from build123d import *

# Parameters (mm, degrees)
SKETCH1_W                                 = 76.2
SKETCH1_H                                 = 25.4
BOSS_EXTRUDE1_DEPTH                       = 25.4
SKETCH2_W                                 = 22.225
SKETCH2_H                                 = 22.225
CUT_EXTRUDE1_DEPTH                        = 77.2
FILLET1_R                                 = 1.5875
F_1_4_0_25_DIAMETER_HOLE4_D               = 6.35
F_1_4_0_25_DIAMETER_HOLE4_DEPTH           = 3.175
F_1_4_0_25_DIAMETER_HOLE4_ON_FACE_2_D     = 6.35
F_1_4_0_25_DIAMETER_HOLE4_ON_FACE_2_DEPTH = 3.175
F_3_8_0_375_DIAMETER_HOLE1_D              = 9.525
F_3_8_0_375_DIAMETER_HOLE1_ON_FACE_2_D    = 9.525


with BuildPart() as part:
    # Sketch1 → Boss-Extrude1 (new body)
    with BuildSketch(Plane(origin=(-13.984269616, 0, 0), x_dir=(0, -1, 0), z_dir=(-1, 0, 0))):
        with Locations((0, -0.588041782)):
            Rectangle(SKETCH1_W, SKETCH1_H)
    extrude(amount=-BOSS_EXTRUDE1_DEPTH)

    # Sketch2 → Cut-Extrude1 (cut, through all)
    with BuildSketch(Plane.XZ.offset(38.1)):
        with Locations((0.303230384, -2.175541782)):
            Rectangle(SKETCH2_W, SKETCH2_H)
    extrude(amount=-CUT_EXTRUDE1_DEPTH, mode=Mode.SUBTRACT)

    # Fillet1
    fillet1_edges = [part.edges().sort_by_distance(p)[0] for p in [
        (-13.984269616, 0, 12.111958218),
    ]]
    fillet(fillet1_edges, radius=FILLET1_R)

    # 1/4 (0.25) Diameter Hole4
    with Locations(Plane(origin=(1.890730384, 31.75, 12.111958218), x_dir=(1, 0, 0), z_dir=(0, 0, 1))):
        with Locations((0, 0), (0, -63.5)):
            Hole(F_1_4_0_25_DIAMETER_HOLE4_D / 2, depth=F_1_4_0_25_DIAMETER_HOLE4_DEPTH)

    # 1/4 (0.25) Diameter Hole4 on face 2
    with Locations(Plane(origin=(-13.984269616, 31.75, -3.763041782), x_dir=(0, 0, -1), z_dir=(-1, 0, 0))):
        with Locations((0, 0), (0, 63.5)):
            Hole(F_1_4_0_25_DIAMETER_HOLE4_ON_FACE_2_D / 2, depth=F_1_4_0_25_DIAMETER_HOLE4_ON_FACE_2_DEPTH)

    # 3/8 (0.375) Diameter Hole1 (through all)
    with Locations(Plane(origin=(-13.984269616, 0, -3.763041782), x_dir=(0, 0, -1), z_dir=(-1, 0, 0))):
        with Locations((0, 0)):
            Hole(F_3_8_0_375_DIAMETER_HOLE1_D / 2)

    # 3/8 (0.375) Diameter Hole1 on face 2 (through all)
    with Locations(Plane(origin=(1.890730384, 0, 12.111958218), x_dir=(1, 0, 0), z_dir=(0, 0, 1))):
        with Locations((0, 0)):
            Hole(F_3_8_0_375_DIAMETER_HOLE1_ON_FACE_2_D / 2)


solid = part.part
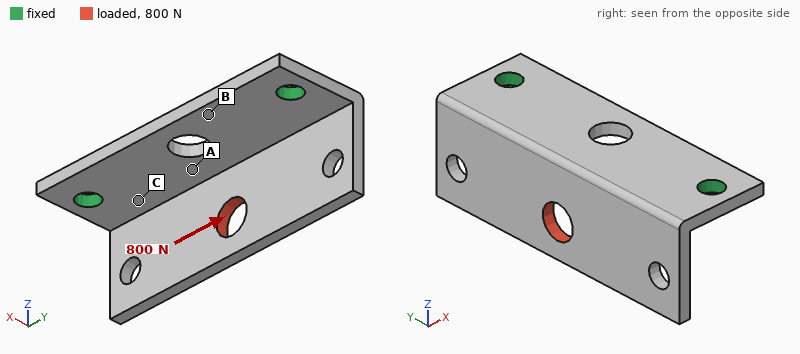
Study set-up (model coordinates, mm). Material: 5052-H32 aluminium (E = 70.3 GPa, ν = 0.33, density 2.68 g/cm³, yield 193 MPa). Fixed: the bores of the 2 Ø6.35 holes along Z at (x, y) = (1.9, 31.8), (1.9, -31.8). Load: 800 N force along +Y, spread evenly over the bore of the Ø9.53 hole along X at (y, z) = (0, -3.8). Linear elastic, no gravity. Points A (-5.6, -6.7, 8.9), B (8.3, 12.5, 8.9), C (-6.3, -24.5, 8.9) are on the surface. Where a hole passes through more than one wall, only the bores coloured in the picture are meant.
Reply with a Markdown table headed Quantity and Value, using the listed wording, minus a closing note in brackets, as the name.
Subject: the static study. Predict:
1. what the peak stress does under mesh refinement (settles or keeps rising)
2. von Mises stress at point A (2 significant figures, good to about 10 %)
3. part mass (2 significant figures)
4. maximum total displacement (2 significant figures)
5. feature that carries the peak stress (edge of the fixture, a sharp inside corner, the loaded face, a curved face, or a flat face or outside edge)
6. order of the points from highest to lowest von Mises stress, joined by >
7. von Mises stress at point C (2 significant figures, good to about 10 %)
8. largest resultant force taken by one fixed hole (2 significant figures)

| Quantity | Value |
|---|---|
| what the peak stress does under mesh refinement | keeps rising |
| von Mises stress at point A | 12 MPa |
| part mass | 28 g |
| maximum total displacement | 57 µm |
| feature that carries the peak stress | edge of the fixture |
| order of the points from highest to lowest von Mises stress, joined by > | C > A > B |
| von Mises stress at point C | 23 MPa |
| largest resultant force taken by one fixed hole | 470 N |
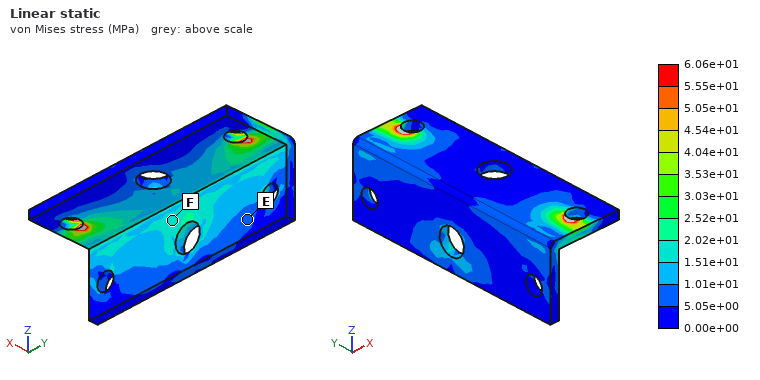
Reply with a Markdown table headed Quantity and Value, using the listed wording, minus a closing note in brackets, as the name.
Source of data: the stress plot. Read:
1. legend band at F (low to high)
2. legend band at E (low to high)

| Quantity | Value |
|---|---|
| legend band at F | 1.51e+01 to 2.02e+01 MPa |
| legend band at E | 5.05e+00 to 1.01e+01 MPa |
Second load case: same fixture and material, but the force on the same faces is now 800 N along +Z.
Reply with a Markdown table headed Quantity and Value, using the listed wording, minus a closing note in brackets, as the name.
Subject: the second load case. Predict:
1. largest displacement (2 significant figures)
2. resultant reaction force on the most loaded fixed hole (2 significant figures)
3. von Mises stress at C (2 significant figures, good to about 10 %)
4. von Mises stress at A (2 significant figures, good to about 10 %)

| Quantity | Value |
|---|---|
| largest displacement | 0.18 mm |
| resultant reaction force on the most loaded fixed hole | 420 N |
| von Mises stress at C | 45 MPa |
| von Mises stress at A | 13 MPa |
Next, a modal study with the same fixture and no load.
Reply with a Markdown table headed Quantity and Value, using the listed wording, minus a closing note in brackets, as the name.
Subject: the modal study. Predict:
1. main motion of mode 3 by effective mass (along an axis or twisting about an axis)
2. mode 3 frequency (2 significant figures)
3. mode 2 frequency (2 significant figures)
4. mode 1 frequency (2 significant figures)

| Quantity | Value |
|---|---|
| main motion of mode 3 by effective mass | along Z |
| mode 3 frequency | 5400 Hz |
| mode 2 frequency | 3800 Hz |
| mode 1 frequency | 2300 Hz |
